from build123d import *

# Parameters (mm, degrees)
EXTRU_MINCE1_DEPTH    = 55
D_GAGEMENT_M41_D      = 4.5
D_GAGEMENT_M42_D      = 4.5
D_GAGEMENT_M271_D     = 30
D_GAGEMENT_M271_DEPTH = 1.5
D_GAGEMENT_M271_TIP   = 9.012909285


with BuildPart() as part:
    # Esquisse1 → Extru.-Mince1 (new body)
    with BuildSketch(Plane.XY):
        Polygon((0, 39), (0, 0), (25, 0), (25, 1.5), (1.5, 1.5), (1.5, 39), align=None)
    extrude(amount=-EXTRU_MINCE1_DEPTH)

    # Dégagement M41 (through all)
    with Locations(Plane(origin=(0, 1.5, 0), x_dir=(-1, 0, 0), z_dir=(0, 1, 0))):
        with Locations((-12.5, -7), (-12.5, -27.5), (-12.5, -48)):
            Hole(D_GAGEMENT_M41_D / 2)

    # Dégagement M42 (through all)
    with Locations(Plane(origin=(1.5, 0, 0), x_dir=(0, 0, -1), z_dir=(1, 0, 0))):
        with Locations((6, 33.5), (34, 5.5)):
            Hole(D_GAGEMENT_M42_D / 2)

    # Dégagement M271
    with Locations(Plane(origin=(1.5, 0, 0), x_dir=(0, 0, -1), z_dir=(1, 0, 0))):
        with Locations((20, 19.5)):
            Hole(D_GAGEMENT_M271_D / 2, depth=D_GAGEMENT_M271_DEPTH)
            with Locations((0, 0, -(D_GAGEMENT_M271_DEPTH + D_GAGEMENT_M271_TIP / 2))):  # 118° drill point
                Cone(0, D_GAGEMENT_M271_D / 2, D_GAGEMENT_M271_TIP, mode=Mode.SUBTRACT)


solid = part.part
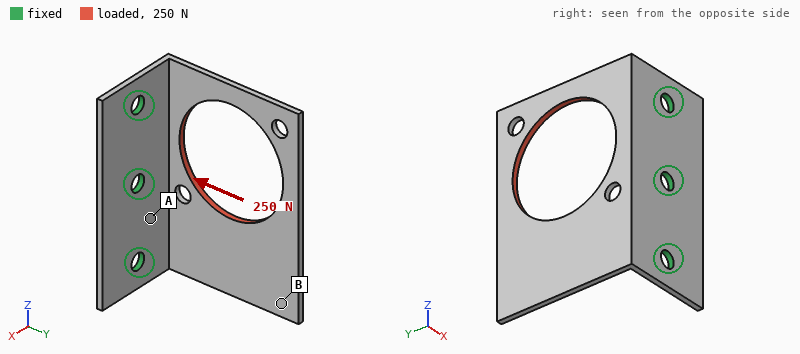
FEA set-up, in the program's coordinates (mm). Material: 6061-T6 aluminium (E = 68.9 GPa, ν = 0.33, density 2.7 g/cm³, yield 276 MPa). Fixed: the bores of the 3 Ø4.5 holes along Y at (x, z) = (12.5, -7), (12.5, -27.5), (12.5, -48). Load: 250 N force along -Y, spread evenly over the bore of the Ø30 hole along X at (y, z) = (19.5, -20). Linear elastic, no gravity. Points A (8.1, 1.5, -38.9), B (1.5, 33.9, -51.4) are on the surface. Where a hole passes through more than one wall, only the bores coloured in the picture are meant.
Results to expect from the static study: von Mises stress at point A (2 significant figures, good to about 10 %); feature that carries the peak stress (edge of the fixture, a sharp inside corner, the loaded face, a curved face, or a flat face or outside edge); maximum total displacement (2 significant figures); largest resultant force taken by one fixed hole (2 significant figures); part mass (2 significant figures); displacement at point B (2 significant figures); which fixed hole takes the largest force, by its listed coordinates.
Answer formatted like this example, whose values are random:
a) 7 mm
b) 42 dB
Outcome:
a) 47 MPa
b) a flat face or outside edge
c) 0.58 mm
d) 130 N
e) 11 g
f) 0.34 mm
g) (12.5, -7)
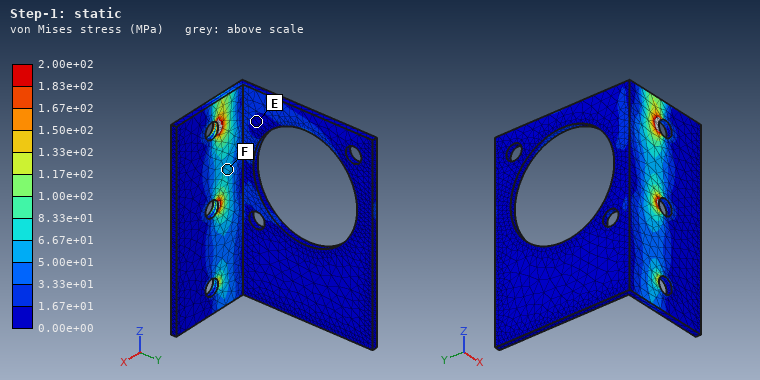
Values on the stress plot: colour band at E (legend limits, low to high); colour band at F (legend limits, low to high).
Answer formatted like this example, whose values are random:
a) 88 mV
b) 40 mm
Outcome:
a) 0.00e+00 to 1.67e+01 MPa
b) 5.00e+01 to 6.67e+01 MPa
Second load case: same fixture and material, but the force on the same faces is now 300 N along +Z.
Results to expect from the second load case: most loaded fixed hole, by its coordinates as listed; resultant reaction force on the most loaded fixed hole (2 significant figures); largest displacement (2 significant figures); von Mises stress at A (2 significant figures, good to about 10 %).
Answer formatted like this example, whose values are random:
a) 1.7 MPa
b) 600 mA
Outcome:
a) (12.5, -7)
b) 190 N
c) 0.44 mm
d) 48 MPa
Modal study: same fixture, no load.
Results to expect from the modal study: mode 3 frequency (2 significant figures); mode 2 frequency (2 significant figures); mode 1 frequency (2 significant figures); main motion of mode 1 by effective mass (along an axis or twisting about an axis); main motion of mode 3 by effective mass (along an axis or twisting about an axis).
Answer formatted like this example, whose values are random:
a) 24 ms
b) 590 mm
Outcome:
a) 2500 Hz
b) 1200 Hz
c) 580 Hz
d) along X
e) along Z
